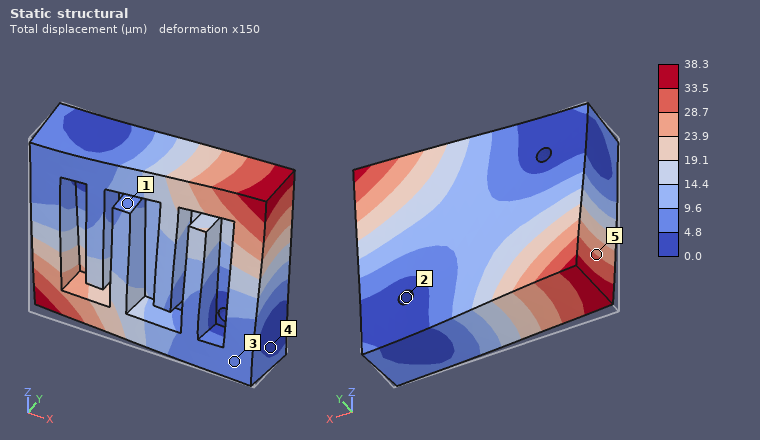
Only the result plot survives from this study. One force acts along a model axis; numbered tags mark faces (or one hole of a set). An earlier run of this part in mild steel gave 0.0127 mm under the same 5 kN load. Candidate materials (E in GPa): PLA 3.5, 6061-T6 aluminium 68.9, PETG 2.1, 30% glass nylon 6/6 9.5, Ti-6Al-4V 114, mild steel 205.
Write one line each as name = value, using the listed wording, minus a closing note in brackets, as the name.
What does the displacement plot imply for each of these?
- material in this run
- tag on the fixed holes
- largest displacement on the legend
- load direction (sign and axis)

material in this run = 6061-T6 aluminium
tag on the fixed holes = 2
largest displacement on the legend = 38.3 µm
load direction = +Y
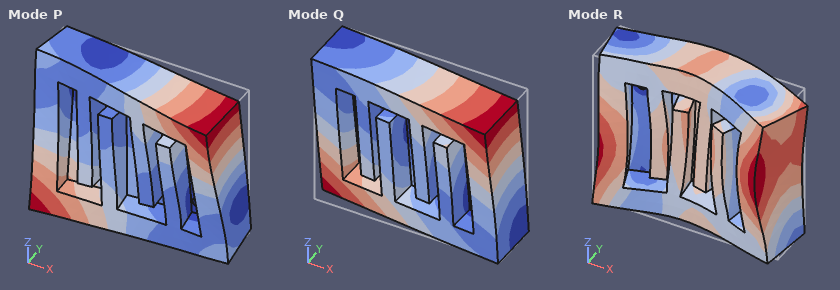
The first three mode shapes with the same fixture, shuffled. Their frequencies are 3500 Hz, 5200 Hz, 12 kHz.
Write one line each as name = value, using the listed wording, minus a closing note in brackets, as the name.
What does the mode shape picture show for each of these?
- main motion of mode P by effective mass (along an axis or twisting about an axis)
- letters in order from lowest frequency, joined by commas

main motion of mode P by effective mass = along Y
letters in order from lowest frequency, joined by commas = Q, P, R
